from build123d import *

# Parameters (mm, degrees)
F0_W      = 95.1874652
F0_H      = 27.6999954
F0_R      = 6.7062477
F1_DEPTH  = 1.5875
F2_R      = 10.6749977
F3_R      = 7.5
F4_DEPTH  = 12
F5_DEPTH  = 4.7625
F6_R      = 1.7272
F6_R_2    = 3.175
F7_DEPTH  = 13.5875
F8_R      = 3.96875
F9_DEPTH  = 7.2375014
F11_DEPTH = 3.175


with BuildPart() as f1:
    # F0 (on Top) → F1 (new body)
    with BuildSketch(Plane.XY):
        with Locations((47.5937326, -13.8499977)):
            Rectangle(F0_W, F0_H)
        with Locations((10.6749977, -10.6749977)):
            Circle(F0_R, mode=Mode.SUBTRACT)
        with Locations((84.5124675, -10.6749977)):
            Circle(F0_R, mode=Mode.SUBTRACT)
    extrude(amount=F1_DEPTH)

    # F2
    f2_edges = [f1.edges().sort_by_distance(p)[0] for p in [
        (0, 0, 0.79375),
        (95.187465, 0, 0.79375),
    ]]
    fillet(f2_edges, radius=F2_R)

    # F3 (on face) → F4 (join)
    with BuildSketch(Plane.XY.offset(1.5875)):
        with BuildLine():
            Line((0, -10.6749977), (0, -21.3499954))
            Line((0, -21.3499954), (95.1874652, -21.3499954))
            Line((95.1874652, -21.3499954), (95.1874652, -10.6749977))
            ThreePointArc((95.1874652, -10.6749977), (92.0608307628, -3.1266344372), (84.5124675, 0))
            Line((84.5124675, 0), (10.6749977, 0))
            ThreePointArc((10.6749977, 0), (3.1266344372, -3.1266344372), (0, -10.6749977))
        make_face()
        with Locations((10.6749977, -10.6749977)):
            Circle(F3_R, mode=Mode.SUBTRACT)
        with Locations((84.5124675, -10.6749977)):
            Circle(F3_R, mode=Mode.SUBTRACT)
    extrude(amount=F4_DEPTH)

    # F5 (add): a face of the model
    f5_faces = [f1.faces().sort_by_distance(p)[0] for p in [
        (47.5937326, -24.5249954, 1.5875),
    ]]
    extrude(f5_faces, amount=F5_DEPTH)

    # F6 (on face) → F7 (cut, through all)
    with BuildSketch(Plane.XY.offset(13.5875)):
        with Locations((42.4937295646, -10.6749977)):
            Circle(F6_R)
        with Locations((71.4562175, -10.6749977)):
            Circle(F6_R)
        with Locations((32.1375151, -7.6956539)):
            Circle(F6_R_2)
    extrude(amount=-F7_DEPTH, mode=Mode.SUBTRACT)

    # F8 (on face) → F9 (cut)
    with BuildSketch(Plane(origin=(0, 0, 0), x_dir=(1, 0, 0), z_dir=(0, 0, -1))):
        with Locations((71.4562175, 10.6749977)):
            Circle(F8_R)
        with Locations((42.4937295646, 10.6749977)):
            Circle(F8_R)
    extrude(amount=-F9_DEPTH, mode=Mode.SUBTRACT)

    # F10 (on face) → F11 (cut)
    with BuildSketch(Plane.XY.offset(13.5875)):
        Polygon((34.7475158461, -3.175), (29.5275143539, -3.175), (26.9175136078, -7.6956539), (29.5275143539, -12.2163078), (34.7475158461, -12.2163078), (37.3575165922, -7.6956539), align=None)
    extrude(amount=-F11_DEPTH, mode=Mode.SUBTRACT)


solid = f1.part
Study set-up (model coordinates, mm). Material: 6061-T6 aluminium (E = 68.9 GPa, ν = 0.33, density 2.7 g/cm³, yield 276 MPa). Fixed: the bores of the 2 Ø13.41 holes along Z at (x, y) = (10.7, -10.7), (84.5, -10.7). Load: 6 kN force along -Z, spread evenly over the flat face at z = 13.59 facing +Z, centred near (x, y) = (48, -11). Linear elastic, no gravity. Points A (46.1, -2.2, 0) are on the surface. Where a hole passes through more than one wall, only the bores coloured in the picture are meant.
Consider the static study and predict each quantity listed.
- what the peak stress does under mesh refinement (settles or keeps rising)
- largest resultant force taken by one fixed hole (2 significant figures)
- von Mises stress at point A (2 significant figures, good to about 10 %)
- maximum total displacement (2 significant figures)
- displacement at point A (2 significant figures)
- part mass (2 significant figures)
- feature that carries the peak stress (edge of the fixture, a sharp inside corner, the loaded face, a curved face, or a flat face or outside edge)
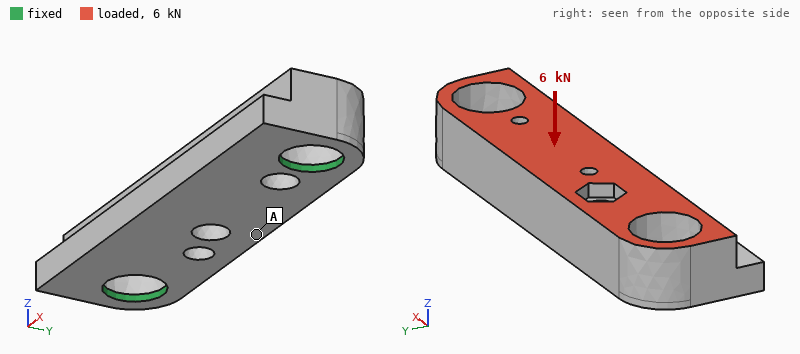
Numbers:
keeps rising
3.7 kN
27 MPa
39 µm
38 µm
67 g
edge of the fixture
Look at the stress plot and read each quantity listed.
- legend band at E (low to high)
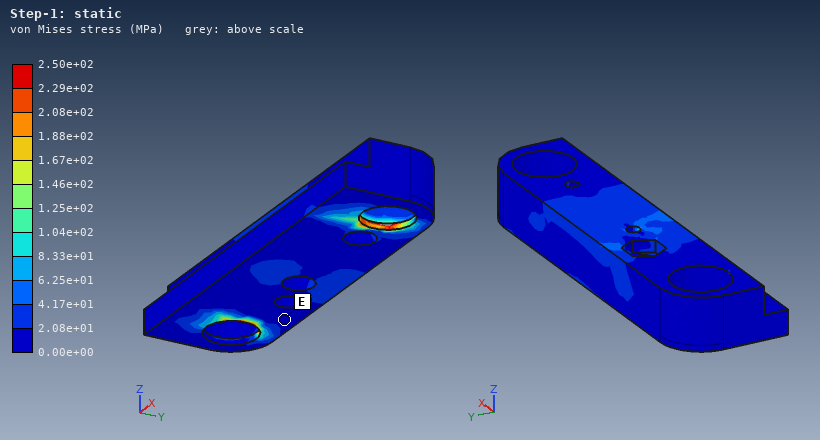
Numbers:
0.00e+00 to 2.08e+01 MPa
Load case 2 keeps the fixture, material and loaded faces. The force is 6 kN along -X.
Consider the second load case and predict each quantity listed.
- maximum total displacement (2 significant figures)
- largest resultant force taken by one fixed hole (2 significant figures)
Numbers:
16 µm
3.3 kN
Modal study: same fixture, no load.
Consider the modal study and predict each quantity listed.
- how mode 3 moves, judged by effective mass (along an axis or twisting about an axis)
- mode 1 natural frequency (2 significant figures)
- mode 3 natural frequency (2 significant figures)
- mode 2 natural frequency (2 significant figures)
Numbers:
along Y
7600 Hz
13 kHz
8800 Hz
